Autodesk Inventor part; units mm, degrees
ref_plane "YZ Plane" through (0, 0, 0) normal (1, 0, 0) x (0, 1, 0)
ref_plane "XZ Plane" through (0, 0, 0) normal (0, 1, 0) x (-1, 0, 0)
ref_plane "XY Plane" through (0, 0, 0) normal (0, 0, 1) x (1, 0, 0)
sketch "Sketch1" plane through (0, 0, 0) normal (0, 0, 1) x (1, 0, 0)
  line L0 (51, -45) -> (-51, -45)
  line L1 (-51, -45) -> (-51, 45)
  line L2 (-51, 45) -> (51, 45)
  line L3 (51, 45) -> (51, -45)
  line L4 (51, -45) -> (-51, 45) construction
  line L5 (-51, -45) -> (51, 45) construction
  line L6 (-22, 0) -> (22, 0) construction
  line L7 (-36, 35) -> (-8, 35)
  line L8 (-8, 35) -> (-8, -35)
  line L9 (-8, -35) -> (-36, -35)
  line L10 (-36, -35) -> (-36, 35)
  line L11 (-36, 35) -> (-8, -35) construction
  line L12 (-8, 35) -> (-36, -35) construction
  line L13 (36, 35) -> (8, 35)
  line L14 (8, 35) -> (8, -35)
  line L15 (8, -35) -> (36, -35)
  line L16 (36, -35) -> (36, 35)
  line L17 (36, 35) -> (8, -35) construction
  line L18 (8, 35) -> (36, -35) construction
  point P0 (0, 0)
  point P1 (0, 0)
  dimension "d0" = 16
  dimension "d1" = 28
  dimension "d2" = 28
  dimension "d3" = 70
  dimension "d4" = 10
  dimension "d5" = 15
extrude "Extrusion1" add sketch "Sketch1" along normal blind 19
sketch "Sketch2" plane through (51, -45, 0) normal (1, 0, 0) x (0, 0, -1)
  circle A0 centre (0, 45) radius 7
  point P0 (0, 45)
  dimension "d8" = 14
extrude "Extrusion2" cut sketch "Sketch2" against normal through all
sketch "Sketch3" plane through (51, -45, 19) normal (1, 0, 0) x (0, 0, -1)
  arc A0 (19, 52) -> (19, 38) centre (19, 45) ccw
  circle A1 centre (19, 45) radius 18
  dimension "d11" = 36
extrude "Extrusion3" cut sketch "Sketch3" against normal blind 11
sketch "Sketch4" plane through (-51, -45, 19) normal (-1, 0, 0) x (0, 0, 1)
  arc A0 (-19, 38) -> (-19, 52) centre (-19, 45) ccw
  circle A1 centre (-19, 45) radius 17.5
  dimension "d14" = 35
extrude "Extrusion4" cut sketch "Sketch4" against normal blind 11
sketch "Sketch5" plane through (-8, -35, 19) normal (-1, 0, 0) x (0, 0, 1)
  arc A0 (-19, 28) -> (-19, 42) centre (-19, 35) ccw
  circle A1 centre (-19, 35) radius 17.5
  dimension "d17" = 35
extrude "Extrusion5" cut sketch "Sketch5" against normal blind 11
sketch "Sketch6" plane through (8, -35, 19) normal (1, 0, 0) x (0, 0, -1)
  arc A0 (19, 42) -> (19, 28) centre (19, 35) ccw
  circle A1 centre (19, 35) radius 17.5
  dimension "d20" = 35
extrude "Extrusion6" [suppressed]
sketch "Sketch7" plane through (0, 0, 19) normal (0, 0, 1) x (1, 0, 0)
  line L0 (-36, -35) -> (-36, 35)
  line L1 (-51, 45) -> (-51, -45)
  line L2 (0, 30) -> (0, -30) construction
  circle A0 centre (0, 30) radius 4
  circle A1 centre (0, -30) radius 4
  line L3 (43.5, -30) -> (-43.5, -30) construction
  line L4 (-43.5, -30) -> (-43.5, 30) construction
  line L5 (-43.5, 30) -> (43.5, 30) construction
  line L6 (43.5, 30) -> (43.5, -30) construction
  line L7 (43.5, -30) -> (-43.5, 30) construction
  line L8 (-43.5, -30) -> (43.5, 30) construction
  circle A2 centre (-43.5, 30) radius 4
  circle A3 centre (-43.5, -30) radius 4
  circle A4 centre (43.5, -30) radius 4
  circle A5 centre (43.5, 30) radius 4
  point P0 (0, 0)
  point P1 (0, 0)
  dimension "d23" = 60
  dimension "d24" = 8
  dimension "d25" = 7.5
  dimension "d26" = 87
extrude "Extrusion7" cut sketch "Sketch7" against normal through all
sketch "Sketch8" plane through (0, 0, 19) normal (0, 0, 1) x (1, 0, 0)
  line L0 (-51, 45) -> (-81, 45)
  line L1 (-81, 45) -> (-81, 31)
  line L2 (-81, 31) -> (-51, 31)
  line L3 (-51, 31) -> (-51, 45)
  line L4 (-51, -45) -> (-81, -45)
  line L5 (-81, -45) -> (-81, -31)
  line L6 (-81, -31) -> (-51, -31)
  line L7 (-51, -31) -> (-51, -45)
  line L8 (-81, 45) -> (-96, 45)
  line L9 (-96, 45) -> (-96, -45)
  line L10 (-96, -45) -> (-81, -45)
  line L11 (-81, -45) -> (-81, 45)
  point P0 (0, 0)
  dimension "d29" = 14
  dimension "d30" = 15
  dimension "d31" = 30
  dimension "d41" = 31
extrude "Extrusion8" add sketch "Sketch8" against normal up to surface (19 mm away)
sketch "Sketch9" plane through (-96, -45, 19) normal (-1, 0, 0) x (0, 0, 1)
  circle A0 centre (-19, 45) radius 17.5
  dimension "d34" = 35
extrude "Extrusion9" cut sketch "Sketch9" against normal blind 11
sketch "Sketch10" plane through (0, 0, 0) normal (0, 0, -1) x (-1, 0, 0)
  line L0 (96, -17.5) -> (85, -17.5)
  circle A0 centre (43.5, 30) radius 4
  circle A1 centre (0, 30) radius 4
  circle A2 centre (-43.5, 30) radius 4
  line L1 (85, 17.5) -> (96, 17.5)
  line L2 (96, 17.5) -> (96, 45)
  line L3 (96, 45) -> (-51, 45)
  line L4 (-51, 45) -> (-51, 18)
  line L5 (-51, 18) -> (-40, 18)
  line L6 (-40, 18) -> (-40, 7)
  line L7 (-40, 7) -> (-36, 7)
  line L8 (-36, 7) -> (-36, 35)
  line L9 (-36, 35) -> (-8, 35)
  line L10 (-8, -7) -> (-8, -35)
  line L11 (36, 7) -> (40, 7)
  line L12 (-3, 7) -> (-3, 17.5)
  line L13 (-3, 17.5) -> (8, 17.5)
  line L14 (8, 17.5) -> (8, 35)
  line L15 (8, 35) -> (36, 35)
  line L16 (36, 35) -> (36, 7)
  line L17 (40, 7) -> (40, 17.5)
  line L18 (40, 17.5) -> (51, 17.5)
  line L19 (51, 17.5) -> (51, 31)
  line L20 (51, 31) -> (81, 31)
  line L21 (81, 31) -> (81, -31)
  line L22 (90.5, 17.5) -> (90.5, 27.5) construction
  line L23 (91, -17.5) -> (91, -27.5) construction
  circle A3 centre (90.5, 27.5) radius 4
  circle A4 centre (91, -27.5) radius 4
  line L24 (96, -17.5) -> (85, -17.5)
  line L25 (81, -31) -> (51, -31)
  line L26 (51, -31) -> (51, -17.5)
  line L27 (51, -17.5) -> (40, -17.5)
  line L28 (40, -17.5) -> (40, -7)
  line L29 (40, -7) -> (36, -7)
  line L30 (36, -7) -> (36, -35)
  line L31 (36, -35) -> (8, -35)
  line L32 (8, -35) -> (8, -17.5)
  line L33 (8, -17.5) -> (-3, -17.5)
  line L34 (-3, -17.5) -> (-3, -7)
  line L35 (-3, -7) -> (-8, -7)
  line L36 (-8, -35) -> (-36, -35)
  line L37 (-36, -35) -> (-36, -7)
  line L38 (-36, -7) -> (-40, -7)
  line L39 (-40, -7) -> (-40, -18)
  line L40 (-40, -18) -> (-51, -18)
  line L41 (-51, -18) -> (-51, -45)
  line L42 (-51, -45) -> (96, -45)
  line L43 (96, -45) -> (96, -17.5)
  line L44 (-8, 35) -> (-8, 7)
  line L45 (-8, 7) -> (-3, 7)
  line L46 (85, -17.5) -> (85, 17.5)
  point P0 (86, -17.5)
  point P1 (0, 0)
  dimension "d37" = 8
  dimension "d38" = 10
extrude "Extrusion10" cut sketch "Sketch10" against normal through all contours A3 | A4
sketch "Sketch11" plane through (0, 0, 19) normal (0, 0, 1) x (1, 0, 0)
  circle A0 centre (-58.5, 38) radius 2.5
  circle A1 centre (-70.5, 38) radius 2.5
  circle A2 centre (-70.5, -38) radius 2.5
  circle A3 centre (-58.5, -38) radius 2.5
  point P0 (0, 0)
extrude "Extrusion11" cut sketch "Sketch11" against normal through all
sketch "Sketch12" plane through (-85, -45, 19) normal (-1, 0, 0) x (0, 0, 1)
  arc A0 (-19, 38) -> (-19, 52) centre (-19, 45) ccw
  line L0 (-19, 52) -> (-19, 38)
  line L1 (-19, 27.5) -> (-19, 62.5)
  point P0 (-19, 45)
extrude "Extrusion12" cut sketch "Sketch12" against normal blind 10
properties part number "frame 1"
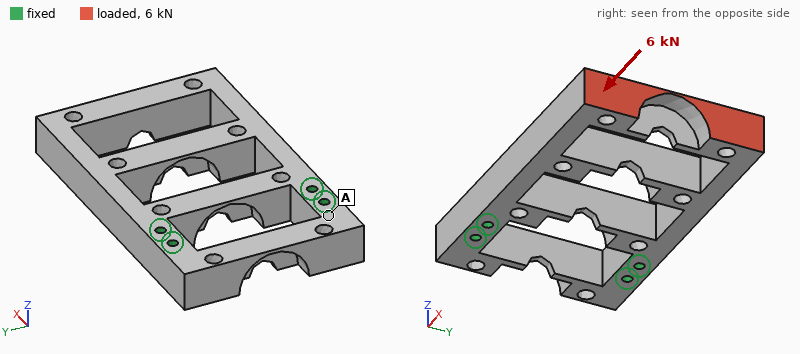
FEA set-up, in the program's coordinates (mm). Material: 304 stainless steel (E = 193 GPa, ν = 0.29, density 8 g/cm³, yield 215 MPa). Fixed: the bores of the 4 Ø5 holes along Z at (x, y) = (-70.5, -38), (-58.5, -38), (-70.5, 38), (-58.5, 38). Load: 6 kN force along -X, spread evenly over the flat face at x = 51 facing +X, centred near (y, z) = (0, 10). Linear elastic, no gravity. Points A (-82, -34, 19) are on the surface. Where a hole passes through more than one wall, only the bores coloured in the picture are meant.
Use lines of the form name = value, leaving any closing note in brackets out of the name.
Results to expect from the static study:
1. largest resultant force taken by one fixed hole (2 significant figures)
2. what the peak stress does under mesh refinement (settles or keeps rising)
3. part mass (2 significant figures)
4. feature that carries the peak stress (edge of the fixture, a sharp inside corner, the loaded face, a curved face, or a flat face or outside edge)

largest resultant force taken by one fixed hole = 2.7 kN
what the peak stress does under mesh refinement = keeps rising
part mass = 880 g
feature that carries the peak stress = a sharp inside corner
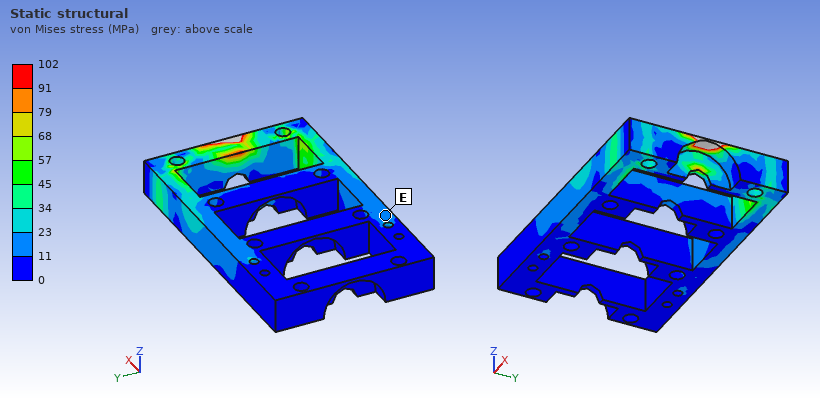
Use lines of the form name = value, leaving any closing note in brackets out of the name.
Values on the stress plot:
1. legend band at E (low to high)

legend band at E = 11 to 23 MPa
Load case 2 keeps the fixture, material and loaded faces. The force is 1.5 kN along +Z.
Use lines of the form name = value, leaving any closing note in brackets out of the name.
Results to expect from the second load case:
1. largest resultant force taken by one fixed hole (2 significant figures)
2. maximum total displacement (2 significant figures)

largest resultant force taken by one fixed hole = 1.2 kN
maximum total displacement = 0.29 mm
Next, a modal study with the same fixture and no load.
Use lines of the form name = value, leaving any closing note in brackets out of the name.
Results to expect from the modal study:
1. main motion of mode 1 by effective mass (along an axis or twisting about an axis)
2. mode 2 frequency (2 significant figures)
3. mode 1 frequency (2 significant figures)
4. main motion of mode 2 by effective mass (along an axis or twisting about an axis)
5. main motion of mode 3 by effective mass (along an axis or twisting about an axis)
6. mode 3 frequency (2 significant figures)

main motion of mode 1 by effective mass = along Z
mode 2 frequency = 1400 Hz
mode 1 frequency = 900 Hz
main motion of mode 2 by effective mass = along Y
main motion of mode 3 by effective mass = along Y
mode 3 frequency = 1700 Hz
